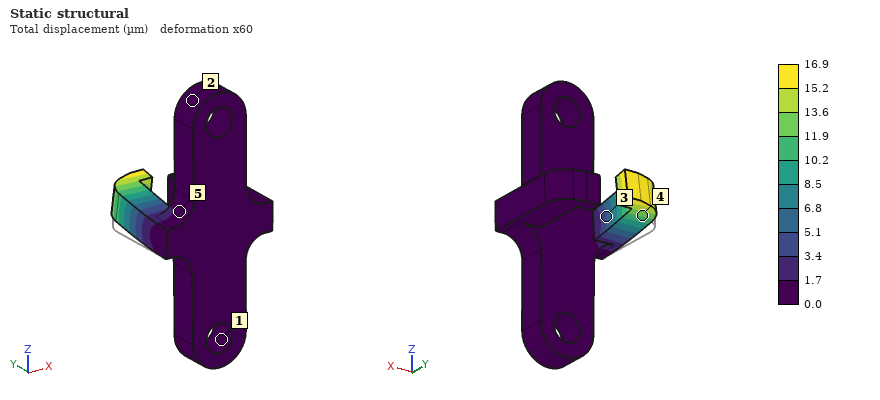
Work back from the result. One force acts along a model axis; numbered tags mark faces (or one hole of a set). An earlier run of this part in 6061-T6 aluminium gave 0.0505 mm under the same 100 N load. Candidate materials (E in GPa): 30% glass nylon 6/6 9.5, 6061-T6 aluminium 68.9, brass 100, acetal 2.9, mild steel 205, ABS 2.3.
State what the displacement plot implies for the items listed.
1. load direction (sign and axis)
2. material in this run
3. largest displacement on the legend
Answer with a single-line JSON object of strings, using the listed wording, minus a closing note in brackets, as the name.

{"load direction": "+Z", "material in this run": "mild steel", "largest displacement on the legend": "16.9 µm"}
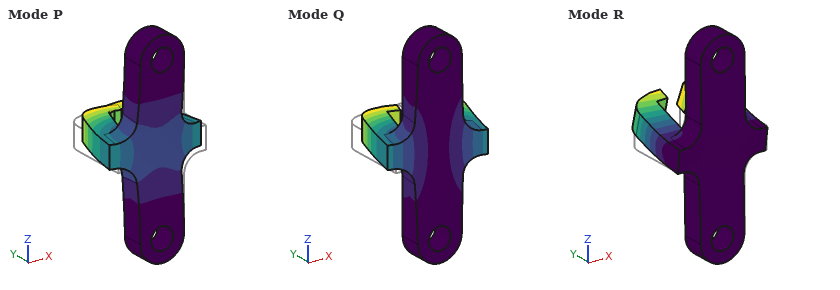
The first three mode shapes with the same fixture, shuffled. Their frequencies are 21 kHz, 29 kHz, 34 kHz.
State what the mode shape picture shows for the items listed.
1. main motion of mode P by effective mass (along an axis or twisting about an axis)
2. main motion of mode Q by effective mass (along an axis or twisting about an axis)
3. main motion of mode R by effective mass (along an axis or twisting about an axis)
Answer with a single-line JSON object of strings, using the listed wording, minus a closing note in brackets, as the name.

{"main motion of mode P by effective mass": "along Y", "main motion of mode Q by effective mass": "along X", "main motion of mode R by effective mass": "along Z"}
